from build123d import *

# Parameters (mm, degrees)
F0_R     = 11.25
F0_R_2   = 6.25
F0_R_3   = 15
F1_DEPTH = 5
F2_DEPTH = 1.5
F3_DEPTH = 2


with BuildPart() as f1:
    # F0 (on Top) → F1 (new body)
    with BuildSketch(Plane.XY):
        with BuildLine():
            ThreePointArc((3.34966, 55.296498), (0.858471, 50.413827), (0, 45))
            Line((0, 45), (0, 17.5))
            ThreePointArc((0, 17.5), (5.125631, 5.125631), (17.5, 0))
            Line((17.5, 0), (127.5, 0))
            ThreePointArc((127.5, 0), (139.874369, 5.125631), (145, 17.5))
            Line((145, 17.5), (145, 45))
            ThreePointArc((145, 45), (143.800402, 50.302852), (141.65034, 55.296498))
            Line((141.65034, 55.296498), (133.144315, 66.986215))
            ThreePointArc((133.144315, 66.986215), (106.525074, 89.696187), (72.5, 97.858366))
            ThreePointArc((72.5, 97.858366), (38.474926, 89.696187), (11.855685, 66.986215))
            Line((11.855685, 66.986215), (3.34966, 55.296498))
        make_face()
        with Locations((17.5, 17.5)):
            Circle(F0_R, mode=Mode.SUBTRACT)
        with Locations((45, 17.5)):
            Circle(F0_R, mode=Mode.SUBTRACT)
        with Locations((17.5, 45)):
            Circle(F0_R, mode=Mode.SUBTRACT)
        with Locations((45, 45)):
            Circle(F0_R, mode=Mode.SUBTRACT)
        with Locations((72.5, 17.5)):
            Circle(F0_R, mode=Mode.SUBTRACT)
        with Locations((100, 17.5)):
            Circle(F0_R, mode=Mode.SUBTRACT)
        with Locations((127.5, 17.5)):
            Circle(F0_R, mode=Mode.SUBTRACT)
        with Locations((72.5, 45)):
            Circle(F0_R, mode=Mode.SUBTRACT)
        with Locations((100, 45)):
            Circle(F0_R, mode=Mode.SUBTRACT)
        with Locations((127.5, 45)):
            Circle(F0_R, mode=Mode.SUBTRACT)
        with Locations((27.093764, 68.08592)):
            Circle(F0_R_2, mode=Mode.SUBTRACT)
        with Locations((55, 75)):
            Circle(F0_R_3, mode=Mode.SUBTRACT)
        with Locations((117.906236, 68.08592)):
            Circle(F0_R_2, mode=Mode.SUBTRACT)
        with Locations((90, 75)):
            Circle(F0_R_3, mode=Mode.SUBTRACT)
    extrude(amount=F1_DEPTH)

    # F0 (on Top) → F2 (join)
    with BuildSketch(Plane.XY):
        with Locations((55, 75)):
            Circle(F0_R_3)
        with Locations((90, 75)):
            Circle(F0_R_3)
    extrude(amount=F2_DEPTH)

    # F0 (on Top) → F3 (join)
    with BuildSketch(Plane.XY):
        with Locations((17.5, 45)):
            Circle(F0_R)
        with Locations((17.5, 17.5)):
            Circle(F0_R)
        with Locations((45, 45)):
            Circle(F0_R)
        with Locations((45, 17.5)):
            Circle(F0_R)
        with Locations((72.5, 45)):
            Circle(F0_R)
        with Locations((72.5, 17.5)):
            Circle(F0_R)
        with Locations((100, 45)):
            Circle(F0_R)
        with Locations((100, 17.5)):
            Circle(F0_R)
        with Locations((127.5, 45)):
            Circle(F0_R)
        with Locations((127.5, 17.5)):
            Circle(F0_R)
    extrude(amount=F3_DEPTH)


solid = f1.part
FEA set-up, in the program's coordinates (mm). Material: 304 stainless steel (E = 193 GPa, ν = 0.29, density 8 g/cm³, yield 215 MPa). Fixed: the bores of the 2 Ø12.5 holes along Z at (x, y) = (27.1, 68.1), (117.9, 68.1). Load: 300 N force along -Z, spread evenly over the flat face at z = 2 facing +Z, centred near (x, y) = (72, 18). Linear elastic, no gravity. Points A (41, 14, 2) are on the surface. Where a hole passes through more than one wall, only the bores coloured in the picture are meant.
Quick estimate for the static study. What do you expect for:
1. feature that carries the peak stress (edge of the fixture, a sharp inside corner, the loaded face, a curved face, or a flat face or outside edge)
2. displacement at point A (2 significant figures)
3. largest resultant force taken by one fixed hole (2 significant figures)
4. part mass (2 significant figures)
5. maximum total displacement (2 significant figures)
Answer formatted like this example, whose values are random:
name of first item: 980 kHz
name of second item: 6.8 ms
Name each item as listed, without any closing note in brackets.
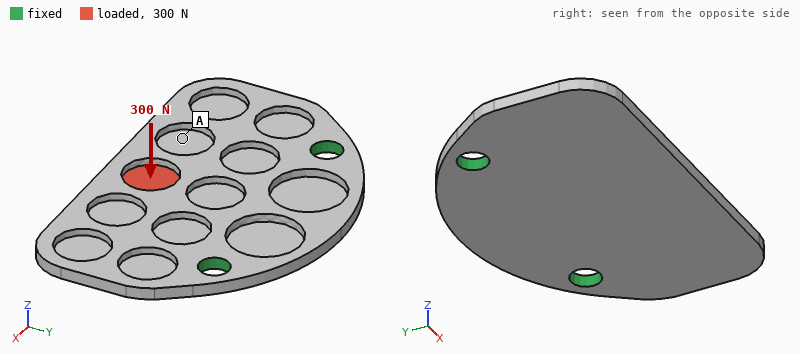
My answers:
feature that carries the peak stress: a curved face
displacement at point A: 0.10 mm
largest resultant force taken by one fixed hole: 160 N
part mass: 340 g
maximum total displacement: 0.17 mm
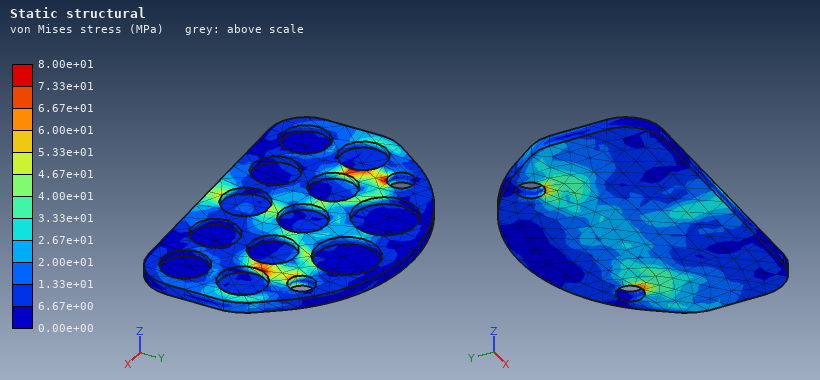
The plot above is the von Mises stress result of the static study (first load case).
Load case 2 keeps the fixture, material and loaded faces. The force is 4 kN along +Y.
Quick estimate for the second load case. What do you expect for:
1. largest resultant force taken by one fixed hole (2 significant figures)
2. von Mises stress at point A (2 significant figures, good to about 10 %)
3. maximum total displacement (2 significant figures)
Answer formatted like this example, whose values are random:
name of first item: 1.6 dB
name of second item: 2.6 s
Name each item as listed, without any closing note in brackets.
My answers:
largest resultant force taken by one fixed hole: 2.1 kN
von Mises stress at point A: 13 MPa
maximum total displacement: 24 µm
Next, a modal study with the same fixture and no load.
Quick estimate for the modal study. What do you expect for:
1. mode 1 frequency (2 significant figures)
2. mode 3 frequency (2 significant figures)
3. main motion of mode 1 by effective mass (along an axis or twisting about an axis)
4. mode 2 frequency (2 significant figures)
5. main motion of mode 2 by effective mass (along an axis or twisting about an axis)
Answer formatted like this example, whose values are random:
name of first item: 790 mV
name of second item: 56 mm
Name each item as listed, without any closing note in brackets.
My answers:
mode 1 frequency: 740 Hz
mode 3 frequency: 1900 Hz
main motion of mode 1 by effective mass: along Z
mode 2 frequency: 1100 Hz
main motion of mode 2 by effective mass: twisting about Y
